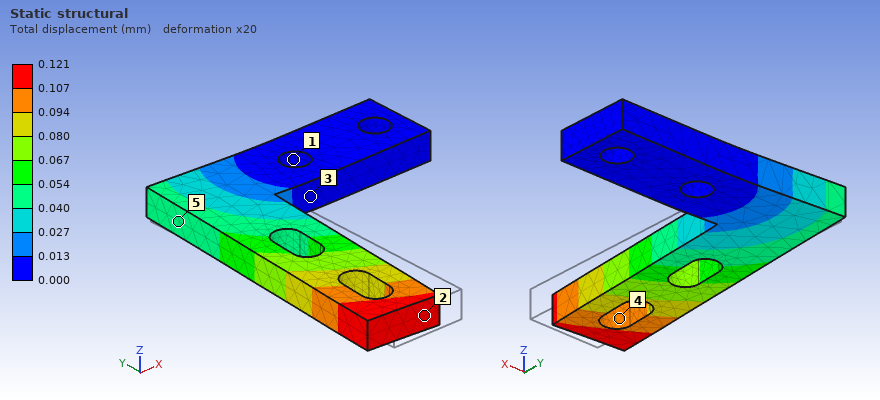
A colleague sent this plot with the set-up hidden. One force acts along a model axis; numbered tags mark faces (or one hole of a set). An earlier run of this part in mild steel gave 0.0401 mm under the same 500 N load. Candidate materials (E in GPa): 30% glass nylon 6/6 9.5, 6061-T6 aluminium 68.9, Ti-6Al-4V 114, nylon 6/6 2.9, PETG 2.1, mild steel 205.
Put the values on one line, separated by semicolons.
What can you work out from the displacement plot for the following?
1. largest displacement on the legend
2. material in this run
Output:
0.121 mm; 6061-T6 aluminium
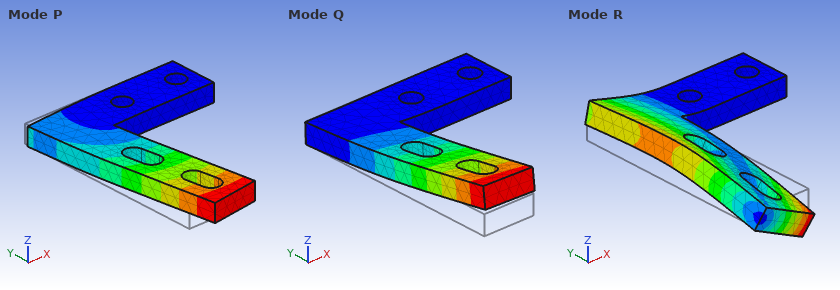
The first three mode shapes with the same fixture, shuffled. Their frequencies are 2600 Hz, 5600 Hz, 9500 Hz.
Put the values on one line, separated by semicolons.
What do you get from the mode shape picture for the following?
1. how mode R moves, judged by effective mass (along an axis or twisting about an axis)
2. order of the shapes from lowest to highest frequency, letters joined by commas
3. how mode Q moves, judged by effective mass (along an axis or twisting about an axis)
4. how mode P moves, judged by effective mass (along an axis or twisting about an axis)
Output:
along Z; Q, P, R; along Z; along X
